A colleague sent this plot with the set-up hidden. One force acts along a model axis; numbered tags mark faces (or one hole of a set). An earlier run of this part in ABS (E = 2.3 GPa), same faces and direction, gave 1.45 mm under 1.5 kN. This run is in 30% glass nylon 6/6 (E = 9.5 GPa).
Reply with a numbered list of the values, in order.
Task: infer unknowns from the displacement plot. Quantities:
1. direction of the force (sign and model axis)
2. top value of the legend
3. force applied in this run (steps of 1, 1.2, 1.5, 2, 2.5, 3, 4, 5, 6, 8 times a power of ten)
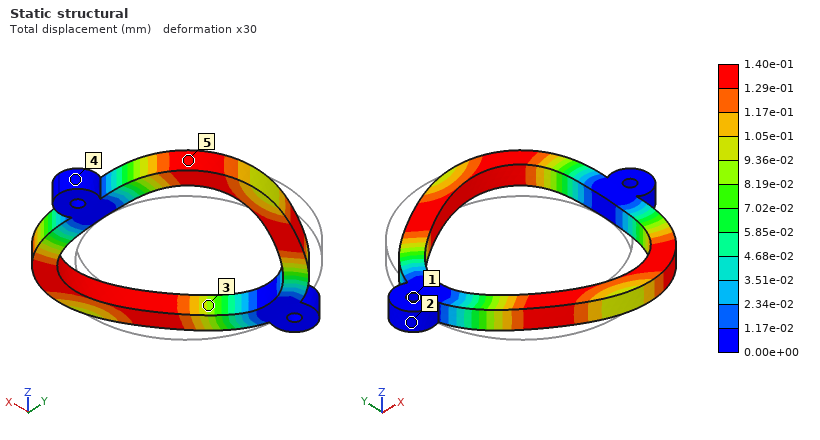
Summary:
1. +X
2. 1.40e-01 mm
3. 600 N
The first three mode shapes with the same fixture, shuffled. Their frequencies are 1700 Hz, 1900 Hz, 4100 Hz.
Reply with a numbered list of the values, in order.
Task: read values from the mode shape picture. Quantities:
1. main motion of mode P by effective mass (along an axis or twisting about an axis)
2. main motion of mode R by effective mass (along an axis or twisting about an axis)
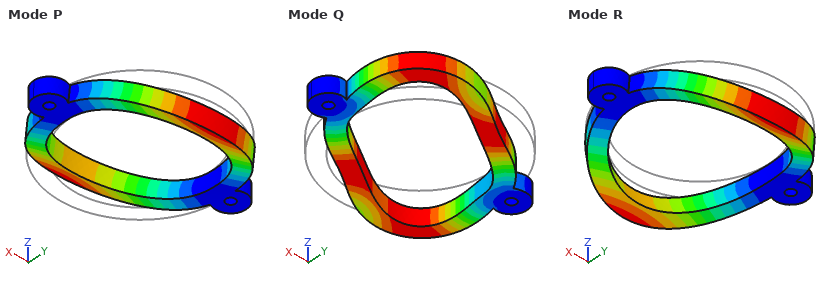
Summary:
1. twisting about X
2. along Z
